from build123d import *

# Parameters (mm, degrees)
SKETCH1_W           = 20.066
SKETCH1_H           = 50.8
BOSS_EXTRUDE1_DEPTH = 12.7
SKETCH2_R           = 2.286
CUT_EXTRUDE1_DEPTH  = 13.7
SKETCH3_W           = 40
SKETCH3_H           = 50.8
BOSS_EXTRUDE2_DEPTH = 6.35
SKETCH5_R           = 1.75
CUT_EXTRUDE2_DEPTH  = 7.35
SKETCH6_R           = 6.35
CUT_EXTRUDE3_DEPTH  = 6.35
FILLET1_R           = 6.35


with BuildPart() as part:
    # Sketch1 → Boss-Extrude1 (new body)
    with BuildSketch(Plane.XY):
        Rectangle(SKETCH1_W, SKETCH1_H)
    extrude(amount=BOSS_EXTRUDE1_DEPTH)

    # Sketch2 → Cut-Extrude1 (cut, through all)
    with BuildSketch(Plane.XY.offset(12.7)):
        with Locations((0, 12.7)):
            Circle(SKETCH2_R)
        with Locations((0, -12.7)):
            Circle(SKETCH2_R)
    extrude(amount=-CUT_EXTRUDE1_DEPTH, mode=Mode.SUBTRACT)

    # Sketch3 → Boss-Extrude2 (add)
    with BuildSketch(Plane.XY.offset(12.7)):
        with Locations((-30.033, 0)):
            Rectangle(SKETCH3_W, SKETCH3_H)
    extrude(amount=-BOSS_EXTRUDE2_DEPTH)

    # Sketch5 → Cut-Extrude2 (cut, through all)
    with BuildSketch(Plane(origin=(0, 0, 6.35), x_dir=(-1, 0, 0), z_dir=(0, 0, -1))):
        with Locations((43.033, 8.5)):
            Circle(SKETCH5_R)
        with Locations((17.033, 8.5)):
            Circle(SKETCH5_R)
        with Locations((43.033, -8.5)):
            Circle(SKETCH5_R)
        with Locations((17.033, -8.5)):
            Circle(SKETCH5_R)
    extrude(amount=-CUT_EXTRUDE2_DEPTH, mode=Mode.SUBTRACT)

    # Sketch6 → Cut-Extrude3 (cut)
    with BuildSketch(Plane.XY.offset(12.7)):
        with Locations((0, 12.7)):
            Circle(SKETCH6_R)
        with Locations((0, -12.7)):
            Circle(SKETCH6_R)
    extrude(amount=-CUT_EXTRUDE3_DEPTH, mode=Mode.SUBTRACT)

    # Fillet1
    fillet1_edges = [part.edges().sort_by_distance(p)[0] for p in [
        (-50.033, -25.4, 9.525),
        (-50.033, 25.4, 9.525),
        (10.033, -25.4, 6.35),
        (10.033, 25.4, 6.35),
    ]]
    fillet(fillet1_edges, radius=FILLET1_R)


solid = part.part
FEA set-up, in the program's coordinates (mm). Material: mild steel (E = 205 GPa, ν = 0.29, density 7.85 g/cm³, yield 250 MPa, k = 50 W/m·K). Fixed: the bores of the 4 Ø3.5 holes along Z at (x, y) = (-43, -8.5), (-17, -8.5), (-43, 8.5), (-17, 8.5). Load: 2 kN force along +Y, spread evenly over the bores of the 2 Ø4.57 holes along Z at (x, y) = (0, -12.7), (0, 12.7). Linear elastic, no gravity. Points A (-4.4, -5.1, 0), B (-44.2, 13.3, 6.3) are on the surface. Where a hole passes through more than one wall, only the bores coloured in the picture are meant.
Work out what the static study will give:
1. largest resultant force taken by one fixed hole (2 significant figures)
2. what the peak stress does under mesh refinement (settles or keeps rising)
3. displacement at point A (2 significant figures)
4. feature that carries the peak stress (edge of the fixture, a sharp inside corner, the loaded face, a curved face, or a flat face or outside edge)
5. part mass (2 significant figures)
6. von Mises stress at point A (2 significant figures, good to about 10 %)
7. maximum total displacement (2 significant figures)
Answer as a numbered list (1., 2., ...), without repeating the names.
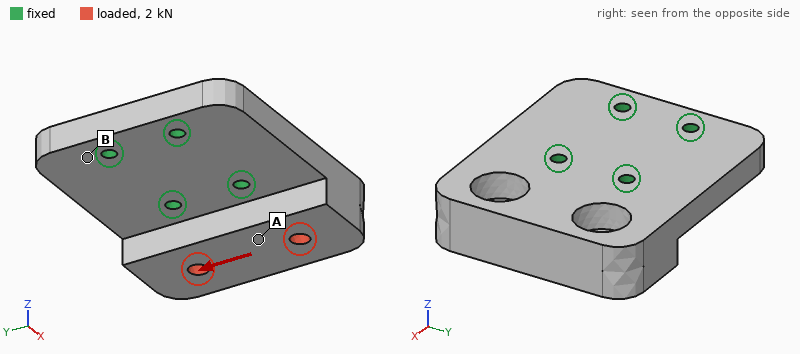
1. 1.6 kN
2. keeps rising
3. 3.2 µm
4. edge of the fixture
5. 180 g
6. 12 MPa
7. 6.0 µm
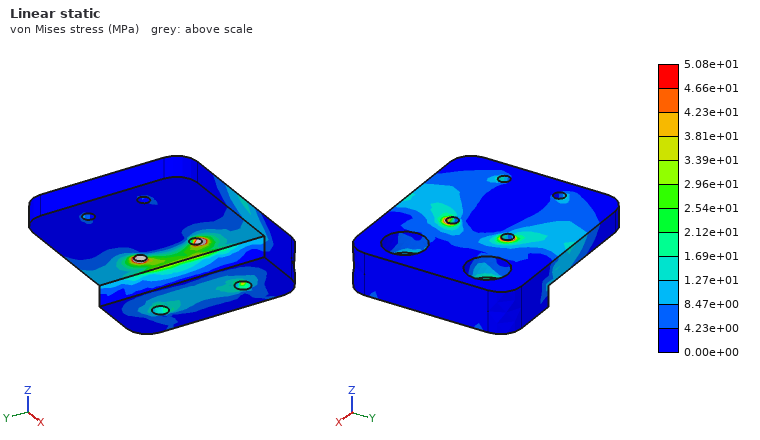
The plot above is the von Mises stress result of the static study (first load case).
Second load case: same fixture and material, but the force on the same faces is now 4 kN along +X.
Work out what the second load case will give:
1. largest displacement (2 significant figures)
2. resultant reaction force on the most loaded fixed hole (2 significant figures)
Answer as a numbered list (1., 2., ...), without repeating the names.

1. 34 µm
2. 1.7 kN
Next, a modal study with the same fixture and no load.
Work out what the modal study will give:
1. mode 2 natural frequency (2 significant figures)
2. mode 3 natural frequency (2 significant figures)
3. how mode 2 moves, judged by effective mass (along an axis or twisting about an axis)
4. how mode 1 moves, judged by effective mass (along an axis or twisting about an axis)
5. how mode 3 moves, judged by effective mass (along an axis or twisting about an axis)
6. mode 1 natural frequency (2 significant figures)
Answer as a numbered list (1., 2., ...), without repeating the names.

1. 8100 Hz
2. 13 kHz
3. twisting about X
4. along Z
5. along Y
6. 4800 Hz
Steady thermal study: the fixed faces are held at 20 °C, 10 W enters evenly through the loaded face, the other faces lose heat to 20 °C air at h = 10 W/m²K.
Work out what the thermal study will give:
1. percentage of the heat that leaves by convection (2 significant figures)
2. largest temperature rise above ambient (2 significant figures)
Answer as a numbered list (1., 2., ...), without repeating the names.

1. 4.7 %
2. 14 K
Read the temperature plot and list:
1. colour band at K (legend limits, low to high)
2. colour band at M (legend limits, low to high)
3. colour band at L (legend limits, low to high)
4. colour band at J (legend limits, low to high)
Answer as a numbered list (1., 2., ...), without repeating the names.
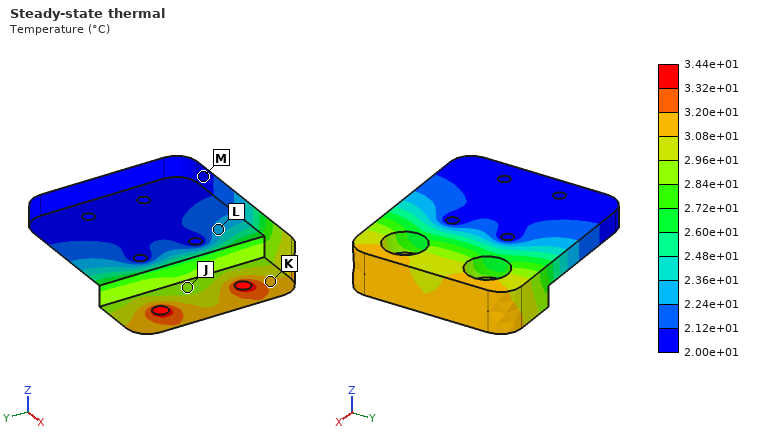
1. 3.08e+01 to 3.20e+01 °C
2. 2.00e+01 to 2.12e+01 °C
3. 2.24e+01 to 2.36e+01 °C
4. 2.84e+01 to 2.96e+01 °C
